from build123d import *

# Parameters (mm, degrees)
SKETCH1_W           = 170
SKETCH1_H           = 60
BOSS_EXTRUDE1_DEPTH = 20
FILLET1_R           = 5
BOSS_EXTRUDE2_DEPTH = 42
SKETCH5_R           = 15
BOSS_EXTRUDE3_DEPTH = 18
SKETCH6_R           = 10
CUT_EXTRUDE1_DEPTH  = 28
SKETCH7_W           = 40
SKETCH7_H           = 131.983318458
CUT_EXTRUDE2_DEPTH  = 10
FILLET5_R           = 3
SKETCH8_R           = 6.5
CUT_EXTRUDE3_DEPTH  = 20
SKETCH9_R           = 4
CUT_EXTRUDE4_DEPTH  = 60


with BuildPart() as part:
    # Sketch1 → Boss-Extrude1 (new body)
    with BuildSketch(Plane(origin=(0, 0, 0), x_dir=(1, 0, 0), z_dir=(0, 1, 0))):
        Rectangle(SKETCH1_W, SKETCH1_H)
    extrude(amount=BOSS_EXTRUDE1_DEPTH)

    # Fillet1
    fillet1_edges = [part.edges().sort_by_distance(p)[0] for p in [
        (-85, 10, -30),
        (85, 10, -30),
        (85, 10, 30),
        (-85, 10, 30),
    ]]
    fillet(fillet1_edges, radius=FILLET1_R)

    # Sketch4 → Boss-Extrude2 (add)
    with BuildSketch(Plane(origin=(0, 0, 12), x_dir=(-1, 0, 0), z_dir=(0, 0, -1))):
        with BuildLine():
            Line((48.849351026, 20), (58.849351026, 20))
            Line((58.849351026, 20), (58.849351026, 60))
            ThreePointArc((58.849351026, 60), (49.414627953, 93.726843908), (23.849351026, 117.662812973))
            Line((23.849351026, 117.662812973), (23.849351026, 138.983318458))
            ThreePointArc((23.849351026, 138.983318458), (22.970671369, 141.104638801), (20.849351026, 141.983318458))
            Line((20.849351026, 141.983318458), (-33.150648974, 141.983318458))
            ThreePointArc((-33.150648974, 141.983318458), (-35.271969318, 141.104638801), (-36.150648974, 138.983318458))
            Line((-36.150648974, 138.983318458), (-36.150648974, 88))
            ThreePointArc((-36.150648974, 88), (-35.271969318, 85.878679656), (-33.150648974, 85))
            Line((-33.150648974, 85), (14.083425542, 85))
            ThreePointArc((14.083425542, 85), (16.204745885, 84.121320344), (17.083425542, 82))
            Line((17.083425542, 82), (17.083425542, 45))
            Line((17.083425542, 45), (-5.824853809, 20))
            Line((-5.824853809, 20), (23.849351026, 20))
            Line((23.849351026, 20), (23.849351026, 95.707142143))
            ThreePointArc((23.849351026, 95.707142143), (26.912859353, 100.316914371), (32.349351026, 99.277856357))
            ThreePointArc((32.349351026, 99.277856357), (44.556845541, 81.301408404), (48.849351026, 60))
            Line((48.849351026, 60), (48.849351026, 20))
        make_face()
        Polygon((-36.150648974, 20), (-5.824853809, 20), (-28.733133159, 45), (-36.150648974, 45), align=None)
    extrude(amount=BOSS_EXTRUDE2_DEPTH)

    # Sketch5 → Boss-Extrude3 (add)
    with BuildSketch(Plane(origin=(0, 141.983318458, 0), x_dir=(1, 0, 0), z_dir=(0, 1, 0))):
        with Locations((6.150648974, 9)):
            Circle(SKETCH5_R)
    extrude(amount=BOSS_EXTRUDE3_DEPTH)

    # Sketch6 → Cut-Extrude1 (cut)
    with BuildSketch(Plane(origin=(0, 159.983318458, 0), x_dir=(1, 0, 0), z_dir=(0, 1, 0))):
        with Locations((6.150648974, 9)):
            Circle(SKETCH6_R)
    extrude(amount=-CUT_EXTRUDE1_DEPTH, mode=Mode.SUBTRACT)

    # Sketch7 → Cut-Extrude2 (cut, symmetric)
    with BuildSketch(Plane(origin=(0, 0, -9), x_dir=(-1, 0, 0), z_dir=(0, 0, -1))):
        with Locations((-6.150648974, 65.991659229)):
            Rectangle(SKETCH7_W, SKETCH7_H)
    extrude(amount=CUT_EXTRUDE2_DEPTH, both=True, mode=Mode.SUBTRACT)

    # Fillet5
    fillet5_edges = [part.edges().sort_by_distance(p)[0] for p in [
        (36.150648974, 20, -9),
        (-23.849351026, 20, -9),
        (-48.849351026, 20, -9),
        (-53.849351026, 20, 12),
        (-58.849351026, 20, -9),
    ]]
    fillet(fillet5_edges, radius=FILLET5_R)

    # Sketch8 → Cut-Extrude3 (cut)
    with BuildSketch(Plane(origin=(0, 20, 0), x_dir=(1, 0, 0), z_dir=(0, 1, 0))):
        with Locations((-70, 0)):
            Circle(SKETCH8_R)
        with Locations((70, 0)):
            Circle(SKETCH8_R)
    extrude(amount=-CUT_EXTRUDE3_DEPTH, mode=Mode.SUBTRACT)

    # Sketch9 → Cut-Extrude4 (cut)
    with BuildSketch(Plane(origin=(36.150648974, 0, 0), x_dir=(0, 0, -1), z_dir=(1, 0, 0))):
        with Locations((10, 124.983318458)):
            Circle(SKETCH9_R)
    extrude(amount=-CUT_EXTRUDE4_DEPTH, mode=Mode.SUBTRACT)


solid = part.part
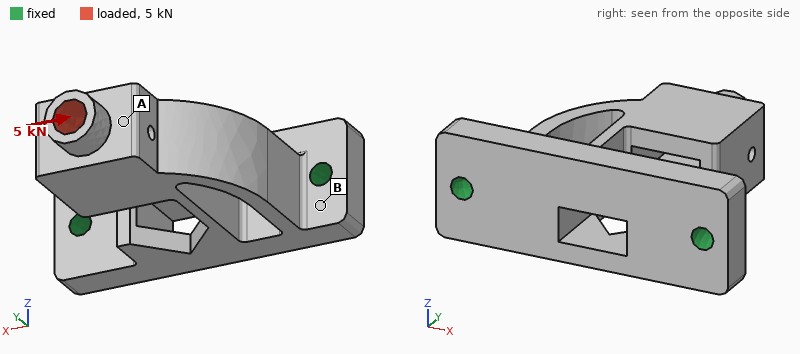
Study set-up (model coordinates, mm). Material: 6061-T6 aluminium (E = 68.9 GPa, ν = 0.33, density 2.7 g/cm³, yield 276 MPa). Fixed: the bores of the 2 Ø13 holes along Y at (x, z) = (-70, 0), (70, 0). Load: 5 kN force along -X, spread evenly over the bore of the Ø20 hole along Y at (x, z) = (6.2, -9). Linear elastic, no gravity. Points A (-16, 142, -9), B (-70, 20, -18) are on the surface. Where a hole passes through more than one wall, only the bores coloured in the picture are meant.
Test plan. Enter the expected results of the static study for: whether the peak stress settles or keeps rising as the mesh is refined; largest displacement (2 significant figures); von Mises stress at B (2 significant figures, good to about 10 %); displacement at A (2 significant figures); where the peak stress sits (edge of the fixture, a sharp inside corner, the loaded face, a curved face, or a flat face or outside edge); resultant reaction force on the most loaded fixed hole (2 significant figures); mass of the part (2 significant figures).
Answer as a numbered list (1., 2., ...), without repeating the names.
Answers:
1. keeps rising
2. 1.1 mm
3. 27 MPa
4. 0.86 mm
5. a sharp inside corner
6. 5.5 kN
7. 1.0 kg
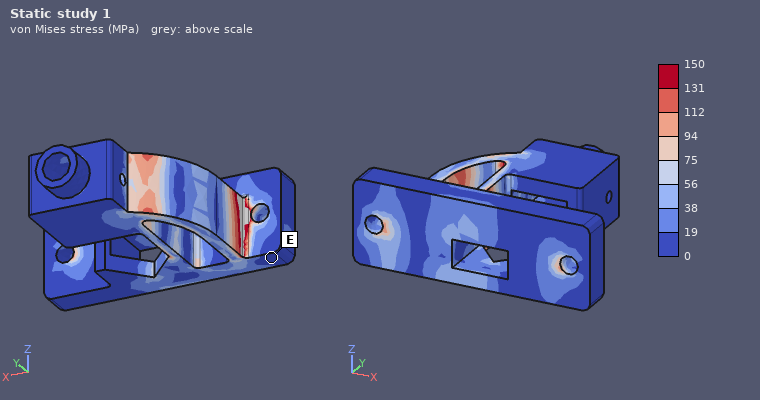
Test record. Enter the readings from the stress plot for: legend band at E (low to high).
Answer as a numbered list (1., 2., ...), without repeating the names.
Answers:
1. 0 to 19 MPa
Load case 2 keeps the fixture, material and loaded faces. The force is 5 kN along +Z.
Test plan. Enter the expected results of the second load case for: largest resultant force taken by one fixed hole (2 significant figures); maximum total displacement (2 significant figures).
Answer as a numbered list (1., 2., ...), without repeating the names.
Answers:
1. 2.7 kN
2. 1.9 mm
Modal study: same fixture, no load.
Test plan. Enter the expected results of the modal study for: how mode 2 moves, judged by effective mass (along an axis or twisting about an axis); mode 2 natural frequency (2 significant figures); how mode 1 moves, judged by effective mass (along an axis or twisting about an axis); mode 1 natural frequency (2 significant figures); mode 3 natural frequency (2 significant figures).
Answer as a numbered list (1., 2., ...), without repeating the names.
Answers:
1. along X
2. 760 Hz
3. along Z
4. 600 Hz
5. 1400 Hz
